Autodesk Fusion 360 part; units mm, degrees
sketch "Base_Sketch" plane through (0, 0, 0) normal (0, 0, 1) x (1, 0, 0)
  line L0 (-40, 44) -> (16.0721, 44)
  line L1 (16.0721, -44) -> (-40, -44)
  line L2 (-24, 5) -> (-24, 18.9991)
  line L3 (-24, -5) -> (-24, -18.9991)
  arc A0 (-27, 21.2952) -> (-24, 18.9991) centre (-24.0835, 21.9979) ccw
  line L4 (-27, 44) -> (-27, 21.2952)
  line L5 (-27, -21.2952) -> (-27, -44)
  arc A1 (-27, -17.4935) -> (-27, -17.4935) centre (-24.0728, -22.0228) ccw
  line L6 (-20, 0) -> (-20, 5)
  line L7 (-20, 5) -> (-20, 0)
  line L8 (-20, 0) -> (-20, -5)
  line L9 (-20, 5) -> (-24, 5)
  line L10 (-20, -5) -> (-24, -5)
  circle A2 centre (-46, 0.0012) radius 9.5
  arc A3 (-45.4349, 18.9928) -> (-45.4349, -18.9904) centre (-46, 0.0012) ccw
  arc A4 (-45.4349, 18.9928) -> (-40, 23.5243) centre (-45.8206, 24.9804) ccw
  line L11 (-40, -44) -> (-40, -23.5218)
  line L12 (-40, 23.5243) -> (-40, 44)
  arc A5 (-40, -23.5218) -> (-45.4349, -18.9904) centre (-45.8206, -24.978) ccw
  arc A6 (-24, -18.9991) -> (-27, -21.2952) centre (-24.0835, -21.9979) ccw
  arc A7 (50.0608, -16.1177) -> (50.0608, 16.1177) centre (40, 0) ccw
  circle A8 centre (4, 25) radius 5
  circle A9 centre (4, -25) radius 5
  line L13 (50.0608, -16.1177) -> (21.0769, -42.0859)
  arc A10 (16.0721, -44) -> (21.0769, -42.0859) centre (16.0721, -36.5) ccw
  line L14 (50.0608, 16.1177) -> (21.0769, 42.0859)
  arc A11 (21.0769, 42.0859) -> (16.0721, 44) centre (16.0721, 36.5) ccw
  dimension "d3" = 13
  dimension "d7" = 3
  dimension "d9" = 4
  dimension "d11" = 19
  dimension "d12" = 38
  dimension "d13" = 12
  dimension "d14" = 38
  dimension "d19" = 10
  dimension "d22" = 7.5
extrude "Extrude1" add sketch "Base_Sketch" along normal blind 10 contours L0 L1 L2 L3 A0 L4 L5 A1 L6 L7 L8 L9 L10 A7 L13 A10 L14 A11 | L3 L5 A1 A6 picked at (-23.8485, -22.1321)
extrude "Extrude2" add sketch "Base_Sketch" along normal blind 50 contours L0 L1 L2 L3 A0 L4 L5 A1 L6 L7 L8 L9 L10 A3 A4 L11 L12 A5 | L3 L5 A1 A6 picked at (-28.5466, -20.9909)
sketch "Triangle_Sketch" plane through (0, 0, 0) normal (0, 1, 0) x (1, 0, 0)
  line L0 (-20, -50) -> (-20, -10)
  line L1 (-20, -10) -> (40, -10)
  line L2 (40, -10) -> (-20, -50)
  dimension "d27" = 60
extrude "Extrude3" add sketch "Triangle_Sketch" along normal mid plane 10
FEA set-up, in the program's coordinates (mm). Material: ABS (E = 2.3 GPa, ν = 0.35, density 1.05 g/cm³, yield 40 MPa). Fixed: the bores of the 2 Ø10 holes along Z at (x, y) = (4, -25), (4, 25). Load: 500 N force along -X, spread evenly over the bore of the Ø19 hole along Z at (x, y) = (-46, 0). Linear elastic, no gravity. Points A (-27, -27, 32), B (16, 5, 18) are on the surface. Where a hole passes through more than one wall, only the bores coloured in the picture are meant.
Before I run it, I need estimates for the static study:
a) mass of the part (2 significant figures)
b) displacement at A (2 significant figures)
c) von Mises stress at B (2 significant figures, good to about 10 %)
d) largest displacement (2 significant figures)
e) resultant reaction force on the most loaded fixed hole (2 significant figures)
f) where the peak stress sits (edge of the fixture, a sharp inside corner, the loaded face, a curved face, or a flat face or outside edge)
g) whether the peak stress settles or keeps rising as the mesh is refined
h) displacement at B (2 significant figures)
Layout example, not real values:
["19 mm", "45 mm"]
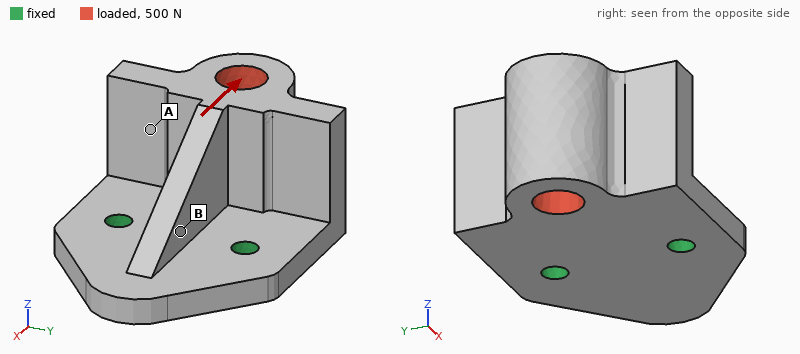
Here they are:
["170 g", "0.20 mm", "1.5 MPa", "0.42 mm", "250 N", "edge of the fixture", "keeps rising", "0.079 mm"]
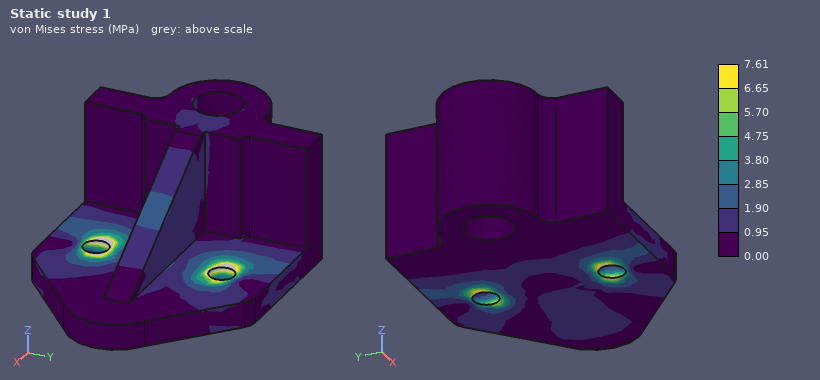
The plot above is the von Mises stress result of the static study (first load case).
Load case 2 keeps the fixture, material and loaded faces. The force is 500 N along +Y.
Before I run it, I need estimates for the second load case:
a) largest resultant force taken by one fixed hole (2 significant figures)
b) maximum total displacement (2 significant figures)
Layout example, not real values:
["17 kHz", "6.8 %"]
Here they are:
["540 N", "0.21 mm"]
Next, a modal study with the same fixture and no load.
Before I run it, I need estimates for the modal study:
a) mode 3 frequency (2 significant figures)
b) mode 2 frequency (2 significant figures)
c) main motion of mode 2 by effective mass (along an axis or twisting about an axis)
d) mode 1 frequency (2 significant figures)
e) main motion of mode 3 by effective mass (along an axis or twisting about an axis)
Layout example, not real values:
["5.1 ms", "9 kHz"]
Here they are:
["1600 Hz", "830 Hz", "along Y", "460 Hz", "along Z"]
